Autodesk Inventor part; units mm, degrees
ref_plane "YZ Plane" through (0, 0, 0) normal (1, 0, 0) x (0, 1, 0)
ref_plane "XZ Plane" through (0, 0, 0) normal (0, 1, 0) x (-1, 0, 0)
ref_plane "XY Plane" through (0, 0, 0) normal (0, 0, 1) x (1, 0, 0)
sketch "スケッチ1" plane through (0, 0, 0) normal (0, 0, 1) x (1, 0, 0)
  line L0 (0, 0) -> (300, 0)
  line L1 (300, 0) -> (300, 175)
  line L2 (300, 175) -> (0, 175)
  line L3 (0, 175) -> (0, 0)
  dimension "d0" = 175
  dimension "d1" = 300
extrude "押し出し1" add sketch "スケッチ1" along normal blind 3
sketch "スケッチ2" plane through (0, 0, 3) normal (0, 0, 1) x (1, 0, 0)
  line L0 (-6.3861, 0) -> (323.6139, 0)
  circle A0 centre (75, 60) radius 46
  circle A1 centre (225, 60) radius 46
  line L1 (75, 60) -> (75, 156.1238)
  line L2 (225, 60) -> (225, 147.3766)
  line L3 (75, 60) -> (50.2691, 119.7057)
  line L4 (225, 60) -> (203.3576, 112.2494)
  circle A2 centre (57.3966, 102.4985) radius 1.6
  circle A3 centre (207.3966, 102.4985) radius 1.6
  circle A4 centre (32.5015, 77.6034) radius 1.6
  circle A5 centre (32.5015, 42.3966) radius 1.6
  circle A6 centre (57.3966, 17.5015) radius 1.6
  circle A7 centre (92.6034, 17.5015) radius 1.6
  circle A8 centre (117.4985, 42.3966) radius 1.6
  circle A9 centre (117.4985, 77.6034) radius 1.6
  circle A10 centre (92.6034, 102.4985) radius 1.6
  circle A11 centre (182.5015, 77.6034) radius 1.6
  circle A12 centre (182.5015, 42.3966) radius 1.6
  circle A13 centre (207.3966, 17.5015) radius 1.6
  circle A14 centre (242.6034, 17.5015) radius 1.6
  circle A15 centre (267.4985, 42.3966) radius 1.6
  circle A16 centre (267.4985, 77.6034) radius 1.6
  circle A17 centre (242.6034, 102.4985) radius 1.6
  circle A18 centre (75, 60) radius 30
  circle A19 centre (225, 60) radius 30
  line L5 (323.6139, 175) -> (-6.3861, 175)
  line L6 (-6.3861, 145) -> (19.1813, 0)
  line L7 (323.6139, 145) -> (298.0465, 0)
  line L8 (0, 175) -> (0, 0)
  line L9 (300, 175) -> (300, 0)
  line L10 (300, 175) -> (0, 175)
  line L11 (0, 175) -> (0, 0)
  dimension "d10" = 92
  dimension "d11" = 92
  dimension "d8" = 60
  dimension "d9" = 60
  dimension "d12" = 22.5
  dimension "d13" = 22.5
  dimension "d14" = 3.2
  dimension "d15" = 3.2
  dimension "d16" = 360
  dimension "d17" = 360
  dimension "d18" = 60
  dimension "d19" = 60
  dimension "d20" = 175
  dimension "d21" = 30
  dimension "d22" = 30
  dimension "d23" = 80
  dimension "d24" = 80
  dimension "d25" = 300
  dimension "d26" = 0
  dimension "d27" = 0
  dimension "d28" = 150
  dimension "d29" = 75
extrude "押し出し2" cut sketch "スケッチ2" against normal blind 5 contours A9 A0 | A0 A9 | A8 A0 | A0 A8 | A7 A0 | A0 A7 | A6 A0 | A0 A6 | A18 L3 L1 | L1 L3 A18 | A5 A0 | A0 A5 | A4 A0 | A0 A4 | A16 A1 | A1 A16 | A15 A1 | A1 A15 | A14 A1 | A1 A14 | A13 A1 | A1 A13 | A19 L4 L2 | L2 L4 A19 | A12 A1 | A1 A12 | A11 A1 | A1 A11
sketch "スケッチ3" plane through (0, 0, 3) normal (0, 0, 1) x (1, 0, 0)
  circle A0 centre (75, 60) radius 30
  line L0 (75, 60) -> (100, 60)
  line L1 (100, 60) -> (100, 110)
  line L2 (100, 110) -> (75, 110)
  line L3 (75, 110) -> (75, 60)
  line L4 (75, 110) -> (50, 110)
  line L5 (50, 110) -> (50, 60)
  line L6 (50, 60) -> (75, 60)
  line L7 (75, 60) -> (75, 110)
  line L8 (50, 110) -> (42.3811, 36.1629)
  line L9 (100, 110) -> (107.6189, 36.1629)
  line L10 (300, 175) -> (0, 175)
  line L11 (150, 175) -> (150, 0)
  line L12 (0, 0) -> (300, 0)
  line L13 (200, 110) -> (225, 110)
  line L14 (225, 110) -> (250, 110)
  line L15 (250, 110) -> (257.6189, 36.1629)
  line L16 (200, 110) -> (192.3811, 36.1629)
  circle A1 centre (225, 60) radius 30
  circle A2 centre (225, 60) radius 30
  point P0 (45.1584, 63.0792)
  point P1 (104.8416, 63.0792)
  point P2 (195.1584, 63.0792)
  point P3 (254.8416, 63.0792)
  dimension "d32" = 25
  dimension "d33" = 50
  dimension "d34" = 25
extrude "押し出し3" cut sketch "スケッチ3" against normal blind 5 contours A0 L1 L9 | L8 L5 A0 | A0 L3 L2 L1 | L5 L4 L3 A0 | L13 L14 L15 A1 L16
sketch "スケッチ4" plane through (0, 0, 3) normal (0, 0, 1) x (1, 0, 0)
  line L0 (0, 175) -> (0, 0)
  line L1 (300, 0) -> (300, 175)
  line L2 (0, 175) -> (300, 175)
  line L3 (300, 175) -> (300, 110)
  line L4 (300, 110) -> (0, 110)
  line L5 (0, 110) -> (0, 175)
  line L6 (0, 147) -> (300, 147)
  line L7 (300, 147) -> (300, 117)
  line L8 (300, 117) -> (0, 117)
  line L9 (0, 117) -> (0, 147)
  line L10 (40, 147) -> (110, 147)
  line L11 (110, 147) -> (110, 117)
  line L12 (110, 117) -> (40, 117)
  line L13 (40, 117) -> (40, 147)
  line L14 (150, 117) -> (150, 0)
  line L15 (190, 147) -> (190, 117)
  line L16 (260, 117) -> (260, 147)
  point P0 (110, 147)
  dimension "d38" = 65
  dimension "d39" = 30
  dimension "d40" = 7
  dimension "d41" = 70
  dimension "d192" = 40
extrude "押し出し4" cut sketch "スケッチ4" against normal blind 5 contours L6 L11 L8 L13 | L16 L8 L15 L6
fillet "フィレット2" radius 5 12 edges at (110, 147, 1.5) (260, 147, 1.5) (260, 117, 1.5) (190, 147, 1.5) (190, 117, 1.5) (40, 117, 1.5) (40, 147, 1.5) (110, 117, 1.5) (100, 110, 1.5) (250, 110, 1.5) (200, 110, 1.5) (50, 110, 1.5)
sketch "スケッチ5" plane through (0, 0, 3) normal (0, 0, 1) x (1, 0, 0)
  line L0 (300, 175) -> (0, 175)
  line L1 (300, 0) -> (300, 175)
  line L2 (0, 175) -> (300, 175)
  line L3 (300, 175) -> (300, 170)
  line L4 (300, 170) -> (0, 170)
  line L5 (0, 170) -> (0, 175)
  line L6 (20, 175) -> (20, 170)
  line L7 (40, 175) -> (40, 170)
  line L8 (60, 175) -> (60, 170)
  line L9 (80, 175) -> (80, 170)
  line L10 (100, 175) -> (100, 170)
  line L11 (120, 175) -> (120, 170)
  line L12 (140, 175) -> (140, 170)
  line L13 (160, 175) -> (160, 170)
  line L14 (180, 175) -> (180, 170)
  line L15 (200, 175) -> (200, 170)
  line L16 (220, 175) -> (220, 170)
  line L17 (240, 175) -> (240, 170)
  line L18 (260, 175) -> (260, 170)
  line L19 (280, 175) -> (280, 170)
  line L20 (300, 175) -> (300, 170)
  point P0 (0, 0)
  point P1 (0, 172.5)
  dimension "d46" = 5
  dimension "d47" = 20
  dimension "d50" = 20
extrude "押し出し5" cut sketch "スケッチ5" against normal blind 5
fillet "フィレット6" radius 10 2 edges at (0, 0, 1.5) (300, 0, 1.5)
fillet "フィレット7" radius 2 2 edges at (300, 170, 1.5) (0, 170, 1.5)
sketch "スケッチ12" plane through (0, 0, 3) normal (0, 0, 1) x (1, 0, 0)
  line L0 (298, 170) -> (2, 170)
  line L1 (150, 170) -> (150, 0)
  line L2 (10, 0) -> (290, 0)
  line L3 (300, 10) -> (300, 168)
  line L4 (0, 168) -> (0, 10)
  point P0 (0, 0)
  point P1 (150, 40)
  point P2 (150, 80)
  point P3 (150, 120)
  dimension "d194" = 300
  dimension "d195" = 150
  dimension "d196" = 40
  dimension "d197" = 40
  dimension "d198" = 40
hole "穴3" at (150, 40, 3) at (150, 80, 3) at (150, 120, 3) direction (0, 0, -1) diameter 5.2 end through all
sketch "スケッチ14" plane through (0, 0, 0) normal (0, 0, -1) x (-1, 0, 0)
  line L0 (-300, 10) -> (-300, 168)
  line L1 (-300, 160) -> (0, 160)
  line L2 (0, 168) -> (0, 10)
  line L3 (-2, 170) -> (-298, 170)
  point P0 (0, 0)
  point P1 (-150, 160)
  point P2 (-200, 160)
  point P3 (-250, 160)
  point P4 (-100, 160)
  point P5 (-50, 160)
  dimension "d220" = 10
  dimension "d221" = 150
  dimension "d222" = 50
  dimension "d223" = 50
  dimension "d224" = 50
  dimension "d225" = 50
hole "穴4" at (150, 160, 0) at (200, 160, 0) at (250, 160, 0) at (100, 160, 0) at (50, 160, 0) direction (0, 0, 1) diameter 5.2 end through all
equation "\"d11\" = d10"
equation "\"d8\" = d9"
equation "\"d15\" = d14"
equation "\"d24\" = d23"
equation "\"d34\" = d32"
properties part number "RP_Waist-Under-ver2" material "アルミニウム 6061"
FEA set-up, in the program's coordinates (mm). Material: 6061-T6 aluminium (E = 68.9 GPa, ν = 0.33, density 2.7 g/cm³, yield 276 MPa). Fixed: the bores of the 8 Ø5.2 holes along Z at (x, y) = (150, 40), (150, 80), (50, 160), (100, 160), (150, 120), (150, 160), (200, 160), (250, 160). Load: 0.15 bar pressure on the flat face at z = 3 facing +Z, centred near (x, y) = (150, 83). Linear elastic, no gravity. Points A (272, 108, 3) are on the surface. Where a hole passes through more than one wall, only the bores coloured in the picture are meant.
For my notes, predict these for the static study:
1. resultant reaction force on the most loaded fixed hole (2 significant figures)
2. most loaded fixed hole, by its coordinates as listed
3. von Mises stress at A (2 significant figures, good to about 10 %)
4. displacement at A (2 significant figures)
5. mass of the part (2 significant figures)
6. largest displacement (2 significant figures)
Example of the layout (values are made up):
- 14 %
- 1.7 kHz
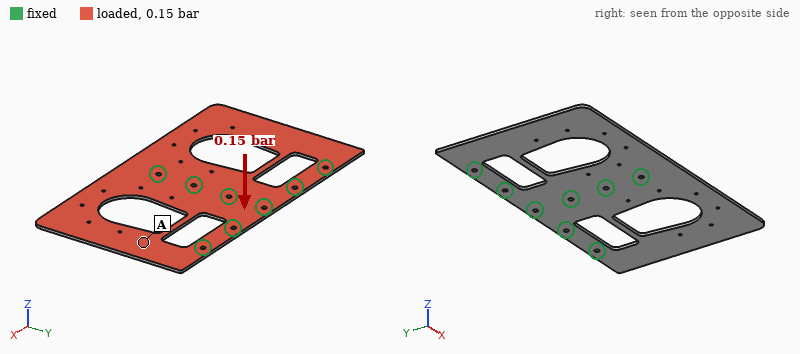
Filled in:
- 260 N
- (150, 40)
- 14 MPa
- 0.96 mm
- 310 g
- 3.5 mm
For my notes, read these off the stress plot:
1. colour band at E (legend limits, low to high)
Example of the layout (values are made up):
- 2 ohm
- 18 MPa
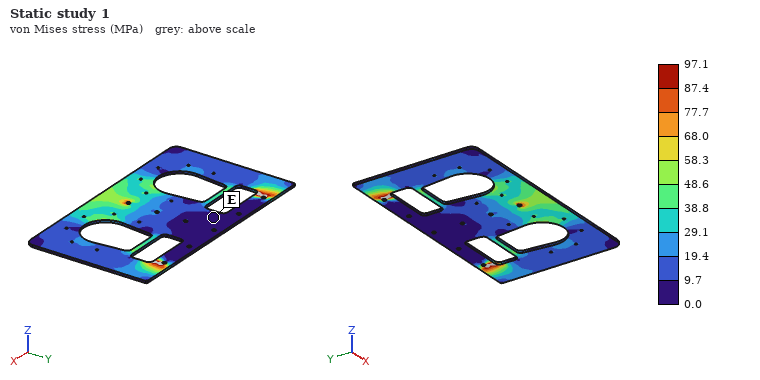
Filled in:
- 0.0 to 9.7 MPa
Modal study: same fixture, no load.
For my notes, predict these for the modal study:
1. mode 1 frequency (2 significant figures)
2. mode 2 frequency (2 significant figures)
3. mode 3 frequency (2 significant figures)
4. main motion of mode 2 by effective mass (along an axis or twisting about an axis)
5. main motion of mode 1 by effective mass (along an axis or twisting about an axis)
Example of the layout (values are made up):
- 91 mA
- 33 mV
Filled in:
- 150 Hz
- 160 Hz
- 480 Hz
- along Z
- twisting about Y
